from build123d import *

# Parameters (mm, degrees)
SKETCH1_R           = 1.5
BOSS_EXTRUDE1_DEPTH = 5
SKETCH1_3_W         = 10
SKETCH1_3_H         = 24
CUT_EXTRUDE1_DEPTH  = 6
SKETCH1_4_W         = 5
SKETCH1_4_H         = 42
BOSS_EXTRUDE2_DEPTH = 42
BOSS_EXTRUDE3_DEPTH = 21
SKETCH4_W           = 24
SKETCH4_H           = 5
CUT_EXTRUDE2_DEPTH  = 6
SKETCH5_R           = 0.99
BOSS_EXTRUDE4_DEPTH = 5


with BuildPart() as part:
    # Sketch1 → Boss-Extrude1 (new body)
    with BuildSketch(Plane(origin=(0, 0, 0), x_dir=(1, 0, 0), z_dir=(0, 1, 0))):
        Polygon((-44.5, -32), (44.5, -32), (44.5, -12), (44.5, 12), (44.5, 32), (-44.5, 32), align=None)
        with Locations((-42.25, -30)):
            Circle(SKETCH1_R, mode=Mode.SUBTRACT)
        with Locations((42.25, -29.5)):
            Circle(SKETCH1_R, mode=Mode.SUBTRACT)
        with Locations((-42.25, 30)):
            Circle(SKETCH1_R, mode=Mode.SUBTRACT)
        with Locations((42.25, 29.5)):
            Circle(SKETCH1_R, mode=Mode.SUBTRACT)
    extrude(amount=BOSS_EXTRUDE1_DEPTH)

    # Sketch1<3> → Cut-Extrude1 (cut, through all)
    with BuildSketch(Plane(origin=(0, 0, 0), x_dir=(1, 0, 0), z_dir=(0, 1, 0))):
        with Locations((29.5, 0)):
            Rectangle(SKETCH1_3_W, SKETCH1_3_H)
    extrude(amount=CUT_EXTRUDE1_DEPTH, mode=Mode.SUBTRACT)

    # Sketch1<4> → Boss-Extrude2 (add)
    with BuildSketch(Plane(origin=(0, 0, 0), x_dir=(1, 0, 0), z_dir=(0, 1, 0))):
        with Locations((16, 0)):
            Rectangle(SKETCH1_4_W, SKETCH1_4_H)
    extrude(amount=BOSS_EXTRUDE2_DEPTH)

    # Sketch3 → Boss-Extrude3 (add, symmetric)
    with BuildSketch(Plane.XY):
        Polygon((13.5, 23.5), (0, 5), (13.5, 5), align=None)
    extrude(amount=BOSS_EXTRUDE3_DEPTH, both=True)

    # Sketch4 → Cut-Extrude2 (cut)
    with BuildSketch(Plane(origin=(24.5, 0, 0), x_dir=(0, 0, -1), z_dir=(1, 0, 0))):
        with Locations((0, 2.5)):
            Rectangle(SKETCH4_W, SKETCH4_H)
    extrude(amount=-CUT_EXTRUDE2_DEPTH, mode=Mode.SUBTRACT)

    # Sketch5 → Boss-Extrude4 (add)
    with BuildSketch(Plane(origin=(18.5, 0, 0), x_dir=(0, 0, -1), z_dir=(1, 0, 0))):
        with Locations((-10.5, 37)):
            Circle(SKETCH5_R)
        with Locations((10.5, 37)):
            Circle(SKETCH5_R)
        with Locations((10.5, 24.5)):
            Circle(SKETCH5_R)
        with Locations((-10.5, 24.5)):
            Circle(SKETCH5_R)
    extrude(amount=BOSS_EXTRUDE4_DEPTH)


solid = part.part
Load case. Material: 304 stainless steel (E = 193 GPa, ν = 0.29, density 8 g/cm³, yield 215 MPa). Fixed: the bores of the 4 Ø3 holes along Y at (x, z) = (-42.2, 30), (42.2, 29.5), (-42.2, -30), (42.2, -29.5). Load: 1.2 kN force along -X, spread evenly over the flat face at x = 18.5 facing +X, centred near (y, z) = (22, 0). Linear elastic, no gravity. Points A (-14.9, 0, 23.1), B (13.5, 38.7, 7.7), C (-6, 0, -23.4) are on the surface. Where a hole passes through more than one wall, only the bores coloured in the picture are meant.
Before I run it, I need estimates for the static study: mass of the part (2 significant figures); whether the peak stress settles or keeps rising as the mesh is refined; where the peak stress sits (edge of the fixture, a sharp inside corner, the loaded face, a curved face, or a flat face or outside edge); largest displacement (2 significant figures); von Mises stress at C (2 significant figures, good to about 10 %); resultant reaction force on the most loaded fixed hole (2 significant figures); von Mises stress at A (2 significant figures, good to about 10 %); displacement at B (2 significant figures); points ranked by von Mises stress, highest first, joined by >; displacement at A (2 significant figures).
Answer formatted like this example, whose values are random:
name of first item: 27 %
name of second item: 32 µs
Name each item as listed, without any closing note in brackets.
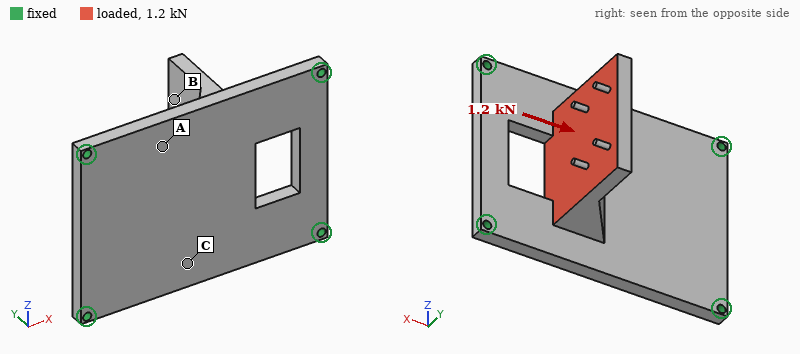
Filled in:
mass of the part: 320 g
whether the peak stress settles or keeps rising as the mesh is refined: keeps rising
where the peak stress sits: edge of the fixture
largest displacement: 51 µm
von Mises stress at C: 25 MPa
resultant reaction force on the most loaded fixed hole: 380 N
von Mises stress at A: 16 MPa
displacement at B: 46 µm
points ranked by von Mises stress, highest first, joined by >: C > A > B
displacement at A: 15 µm
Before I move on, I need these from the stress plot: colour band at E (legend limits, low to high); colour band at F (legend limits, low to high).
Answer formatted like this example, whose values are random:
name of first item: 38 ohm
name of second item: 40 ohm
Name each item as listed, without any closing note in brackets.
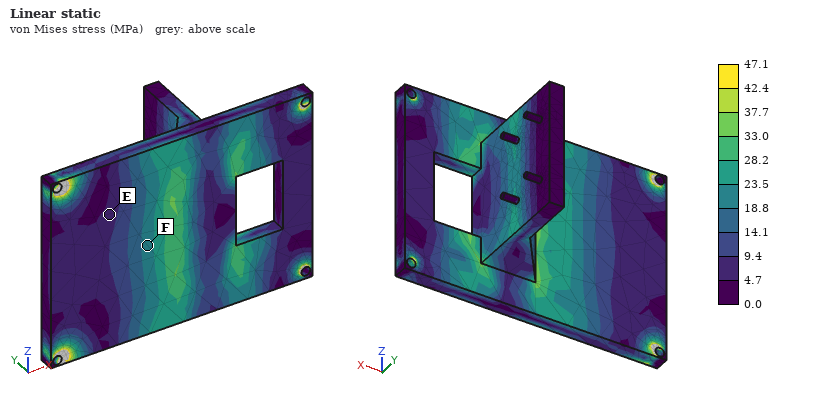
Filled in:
colour band at E: 4.7 to 9.4 MPa
colour band at F: 18.8 to 23.5 MPa
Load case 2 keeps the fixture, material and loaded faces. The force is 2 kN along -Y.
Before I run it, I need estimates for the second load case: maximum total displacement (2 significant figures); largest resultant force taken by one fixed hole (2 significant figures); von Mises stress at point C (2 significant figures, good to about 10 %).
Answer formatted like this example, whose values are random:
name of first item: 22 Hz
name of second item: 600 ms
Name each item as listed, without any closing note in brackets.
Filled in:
maximum total displacement: 64 µm
largest resultant force taken by one fixed hole: 790 N
von Mises stress at point C: 28 MPa
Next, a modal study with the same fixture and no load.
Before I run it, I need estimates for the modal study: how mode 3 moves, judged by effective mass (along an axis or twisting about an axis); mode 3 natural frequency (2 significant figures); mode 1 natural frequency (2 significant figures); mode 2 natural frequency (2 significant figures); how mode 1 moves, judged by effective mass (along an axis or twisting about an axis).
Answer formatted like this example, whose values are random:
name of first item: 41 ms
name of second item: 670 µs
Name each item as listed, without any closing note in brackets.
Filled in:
how mode 3 moves, judged by effective mass: along X
mode 3 natural frequency: 3300 Hz
mode 1 natural frequency: 2000 Hz
mode 2 natural frequency: 2800 Hz
how mode 1 moves, judged by effective mass: along Y
